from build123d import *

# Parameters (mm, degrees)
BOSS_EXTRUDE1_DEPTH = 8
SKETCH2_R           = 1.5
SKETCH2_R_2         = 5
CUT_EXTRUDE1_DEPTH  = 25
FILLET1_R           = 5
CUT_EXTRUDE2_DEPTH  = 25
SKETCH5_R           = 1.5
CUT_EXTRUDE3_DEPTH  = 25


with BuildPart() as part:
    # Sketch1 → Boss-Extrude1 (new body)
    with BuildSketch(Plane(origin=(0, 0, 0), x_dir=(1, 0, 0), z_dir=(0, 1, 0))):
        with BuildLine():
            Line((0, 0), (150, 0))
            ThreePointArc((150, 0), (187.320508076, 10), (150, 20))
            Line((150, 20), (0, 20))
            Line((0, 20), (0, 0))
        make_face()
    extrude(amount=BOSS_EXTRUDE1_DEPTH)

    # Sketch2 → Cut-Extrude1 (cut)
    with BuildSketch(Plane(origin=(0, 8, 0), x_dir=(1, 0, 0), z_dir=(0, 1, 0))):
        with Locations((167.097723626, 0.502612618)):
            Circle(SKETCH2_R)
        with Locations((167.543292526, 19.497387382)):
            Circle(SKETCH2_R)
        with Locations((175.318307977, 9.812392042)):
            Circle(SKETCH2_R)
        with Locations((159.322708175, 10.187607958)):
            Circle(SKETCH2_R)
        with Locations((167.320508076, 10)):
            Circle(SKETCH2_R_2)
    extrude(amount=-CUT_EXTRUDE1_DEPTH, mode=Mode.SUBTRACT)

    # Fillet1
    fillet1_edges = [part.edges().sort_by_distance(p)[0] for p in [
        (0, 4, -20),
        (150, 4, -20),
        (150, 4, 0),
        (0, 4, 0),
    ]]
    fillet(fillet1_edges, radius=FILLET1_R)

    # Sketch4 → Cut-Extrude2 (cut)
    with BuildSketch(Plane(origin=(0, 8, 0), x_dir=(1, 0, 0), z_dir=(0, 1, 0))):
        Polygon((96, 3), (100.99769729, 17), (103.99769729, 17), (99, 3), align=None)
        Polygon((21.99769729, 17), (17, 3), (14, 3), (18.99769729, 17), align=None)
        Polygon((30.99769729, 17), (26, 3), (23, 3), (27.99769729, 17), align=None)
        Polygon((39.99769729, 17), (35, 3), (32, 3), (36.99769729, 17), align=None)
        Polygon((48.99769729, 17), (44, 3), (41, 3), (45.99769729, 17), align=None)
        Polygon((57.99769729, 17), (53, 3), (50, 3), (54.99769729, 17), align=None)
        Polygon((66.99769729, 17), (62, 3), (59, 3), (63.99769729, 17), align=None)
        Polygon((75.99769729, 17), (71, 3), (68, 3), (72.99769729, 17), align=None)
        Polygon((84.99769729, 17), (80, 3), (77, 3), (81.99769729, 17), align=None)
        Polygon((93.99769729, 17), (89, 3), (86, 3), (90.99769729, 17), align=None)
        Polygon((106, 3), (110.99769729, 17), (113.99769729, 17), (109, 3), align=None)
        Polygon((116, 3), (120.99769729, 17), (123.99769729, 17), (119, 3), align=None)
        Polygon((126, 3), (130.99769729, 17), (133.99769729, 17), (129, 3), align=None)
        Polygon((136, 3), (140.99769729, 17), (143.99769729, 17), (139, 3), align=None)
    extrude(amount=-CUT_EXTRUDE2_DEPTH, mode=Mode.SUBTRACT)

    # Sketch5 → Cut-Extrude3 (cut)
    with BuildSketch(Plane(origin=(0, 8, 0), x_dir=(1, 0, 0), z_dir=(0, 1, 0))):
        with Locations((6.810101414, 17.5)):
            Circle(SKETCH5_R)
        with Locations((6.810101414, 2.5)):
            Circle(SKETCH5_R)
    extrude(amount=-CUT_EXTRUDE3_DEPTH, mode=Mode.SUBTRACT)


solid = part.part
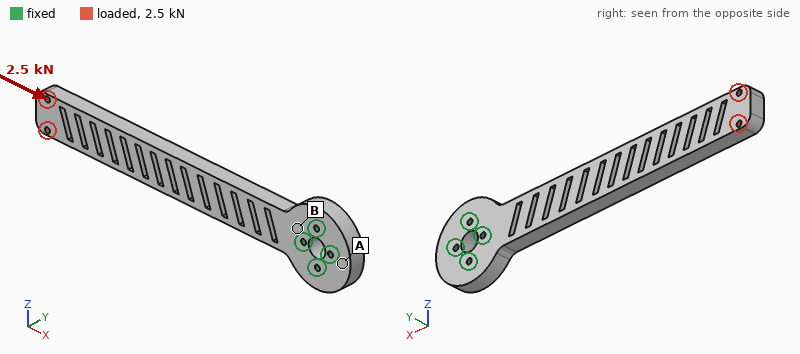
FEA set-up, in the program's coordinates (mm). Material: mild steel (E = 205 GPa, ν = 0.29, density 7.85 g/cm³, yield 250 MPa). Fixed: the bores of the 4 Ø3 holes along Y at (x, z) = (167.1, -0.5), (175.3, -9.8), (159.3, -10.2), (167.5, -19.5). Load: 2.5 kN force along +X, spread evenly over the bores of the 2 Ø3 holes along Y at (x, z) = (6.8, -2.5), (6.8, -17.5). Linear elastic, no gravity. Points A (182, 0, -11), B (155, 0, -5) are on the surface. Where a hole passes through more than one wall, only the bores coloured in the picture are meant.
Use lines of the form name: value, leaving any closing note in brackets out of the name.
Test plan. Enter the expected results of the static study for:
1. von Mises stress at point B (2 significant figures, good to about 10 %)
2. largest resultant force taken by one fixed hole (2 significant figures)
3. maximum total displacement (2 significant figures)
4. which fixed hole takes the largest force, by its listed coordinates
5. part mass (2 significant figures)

von Mises stress at point B: 12 MPa
largest resultant force taken by one fixed hole: 1.2 kN
maximum total displacement: 34 µm
which fixed hole takes the largest force, by its listed coordinates: (159.3, -10.2)
part mass: 220 g
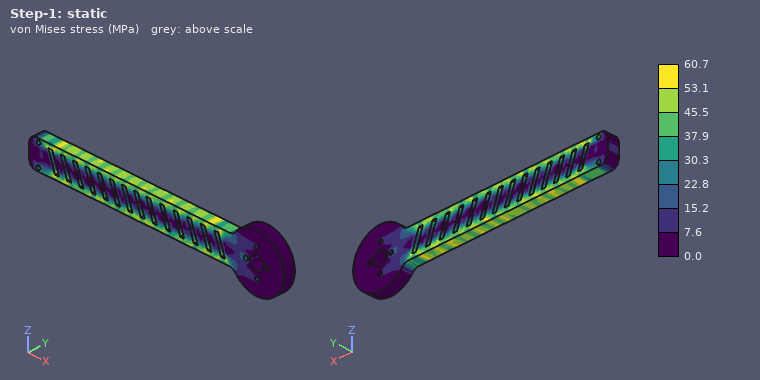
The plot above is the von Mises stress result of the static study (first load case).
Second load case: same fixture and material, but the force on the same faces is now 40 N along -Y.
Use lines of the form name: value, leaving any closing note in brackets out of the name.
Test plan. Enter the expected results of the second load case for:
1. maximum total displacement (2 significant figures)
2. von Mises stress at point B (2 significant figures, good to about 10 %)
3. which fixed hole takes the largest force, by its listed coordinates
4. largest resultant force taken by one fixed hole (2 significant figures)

maximum total displacement: 0.68 mm
von Mises stress at point B: 18 MPa
which fixed hole takes the largest force, by its listed coordinates: (159.3, -10.2)
largest resultant force taken by one fixed hole: 260 N
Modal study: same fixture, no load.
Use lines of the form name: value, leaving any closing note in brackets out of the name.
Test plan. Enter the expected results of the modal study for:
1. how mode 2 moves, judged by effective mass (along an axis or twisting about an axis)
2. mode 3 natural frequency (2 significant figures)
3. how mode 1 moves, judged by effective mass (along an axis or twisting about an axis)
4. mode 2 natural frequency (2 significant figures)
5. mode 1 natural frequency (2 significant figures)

how mode 2 moves, judged by effective mass: along Z
mode 3 natural frequency: 1200 Hz
how mode 1 moves, judged by effective mass: along Y
mode 2 natural frequency: 620 Hz
mode 1 natural frequency: 190 Hz
